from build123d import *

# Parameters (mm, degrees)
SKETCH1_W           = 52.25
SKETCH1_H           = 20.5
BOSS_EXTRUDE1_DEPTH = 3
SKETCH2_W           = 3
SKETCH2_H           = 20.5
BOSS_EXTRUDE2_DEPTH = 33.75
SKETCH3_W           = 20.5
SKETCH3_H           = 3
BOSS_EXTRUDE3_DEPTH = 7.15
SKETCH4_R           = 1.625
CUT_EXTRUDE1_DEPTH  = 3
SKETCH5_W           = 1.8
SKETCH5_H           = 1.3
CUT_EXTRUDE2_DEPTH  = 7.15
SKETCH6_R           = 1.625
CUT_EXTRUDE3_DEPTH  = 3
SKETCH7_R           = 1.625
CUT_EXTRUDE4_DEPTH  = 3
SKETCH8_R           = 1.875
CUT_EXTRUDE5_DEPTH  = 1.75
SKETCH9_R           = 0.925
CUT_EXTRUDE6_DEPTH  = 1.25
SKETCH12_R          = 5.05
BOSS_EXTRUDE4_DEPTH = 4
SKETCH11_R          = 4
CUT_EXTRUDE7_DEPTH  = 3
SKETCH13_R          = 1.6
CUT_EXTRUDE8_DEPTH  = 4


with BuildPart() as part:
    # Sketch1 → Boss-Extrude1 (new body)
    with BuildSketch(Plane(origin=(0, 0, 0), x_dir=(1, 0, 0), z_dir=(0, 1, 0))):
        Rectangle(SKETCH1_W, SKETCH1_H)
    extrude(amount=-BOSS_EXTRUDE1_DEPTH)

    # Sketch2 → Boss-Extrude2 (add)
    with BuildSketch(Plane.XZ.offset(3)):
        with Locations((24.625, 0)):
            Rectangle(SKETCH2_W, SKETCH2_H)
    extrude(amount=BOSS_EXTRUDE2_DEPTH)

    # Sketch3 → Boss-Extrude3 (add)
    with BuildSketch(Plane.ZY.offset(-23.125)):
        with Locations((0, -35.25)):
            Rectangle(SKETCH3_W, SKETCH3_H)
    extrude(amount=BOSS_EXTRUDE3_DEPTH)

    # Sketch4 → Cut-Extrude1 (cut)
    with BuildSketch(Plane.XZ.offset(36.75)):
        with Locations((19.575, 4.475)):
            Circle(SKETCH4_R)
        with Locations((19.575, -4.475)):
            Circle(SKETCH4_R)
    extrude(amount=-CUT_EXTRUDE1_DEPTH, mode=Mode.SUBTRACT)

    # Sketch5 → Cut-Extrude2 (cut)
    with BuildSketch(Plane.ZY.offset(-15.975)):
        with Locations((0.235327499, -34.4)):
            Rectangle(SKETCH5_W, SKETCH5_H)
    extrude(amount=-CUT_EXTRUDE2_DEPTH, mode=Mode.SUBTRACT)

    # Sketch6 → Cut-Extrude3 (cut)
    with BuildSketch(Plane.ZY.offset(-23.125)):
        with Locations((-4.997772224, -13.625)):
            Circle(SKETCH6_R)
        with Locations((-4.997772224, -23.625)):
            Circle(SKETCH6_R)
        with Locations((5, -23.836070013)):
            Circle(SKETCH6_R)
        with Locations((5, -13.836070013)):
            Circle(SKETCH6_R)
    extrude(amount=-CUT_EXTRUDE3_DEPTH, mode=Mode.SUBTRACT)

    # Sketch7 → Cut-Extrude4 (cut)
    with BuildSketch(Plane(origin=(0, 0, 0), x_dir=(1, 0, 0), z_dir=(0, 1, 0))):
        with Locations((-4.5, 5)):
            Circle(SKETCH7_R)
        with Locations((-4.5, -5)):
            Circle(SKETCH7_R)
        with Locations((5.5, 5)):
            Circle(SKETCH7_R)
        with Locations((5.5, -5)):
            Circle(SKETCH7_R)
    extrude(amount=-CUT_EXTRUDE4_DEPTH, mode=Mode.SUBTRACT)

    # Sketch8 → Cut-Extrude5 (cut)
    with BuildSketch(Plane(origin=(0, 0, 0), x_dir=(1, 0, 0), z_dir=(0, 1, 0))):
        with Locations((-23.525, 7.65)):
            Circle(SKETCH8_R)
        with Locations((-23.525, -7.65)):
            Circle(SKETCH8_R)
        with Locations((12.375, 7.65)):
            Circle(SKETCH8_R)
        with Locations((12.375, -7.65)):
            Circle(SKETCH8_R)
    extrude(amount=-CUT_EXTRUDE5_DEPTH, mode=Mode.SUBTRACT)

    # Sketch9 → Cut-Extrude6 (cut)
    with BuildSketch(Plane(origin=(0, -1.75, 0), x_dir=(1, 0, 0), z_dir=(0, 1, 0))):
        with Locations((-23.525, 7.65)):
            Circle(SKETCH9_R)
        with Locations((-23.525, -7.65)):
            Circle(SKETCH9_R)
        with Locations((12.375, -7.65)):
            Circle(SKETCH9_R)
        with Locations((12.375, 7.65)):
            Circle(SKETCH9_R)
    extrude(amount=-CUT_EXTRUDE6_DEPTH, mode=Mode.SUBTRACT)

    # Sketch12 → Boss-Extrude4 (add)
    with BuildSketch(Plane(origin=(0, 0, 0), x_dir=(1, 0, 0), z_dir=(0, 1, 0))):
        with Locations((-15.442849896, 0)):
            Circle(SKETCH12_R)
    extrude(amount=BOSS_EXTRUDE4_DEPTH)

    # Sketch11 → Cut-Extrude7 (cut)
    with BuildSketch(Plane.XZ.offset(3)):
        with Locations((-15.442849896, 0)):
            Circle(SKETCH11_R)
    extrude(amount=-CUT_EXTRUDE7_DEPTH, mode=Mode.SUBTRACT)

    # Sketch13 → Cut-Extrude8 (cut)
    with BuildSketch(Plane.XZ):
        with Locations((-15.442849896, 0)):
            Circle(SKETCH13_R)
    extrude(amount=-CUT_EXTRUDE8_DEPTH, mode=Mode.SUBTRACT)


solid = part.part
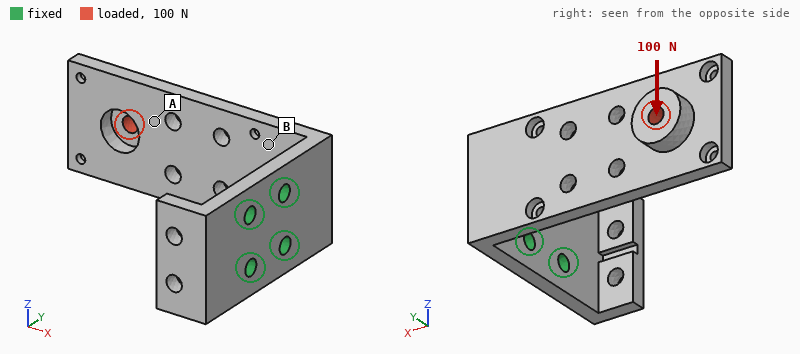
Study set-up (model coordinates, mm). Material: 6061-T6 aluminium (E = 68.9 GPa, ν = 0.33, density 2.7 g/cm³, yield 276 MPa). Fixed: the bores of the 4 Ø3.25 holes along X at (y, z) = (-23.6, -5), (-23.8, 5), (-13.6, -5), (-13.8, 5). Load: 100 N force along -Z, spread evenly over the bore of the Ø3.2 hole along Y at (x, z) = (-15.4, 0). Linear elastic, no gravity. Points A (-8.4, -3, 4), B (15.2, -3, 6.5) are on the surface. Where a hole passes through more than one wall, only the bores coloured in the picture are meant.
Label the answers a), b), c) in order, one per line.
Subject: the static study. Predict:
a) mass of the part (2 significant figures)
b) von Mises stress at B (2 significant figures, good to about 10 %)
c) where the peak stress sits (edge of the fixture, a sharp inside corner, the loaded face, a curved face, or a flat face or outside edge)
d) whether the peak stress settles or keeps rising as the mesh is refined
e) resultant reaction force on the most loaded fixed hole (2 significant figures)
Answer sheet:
a) 15 g
b) 20 MPa
c) edge of the fixture
d) keeps rising
e) 330 N
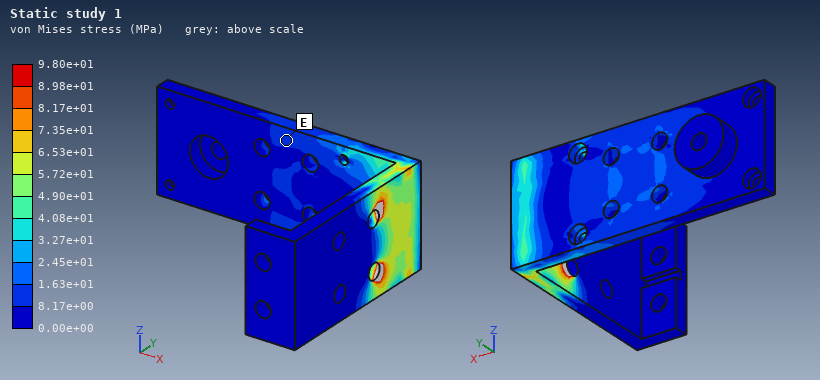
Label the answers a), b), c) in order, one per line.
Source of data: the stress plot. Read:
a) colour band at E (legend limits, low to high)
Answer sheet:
a) 8.17e+00 to 1.63e+01 MPa
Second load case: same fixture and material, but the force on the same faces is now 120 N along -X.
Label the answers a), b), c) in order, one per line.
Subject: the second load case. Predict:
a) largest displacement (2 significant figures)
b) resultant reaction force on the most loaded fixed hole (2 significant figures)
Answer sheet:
a) 0.37 mm
b) 76 N
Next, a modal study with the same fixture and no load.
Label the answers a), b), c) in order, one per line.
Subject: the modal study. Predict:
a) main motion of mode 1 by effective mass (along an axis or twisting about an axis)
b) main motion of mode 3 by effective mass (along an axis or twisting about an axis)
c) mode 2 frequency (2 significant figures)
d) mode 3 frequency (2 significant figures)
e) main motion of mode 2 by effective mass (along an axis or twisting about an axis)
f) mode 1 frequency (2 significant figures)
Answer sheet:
a) along Y
b) along X
c) 1600 Hz
d) 4100 Hz
e) along Z
f) 680 Hz
